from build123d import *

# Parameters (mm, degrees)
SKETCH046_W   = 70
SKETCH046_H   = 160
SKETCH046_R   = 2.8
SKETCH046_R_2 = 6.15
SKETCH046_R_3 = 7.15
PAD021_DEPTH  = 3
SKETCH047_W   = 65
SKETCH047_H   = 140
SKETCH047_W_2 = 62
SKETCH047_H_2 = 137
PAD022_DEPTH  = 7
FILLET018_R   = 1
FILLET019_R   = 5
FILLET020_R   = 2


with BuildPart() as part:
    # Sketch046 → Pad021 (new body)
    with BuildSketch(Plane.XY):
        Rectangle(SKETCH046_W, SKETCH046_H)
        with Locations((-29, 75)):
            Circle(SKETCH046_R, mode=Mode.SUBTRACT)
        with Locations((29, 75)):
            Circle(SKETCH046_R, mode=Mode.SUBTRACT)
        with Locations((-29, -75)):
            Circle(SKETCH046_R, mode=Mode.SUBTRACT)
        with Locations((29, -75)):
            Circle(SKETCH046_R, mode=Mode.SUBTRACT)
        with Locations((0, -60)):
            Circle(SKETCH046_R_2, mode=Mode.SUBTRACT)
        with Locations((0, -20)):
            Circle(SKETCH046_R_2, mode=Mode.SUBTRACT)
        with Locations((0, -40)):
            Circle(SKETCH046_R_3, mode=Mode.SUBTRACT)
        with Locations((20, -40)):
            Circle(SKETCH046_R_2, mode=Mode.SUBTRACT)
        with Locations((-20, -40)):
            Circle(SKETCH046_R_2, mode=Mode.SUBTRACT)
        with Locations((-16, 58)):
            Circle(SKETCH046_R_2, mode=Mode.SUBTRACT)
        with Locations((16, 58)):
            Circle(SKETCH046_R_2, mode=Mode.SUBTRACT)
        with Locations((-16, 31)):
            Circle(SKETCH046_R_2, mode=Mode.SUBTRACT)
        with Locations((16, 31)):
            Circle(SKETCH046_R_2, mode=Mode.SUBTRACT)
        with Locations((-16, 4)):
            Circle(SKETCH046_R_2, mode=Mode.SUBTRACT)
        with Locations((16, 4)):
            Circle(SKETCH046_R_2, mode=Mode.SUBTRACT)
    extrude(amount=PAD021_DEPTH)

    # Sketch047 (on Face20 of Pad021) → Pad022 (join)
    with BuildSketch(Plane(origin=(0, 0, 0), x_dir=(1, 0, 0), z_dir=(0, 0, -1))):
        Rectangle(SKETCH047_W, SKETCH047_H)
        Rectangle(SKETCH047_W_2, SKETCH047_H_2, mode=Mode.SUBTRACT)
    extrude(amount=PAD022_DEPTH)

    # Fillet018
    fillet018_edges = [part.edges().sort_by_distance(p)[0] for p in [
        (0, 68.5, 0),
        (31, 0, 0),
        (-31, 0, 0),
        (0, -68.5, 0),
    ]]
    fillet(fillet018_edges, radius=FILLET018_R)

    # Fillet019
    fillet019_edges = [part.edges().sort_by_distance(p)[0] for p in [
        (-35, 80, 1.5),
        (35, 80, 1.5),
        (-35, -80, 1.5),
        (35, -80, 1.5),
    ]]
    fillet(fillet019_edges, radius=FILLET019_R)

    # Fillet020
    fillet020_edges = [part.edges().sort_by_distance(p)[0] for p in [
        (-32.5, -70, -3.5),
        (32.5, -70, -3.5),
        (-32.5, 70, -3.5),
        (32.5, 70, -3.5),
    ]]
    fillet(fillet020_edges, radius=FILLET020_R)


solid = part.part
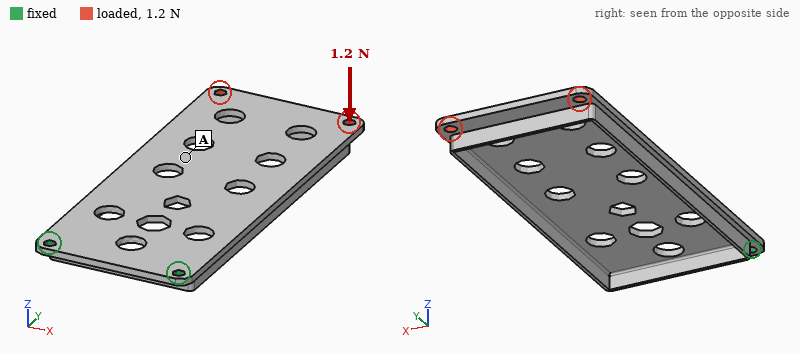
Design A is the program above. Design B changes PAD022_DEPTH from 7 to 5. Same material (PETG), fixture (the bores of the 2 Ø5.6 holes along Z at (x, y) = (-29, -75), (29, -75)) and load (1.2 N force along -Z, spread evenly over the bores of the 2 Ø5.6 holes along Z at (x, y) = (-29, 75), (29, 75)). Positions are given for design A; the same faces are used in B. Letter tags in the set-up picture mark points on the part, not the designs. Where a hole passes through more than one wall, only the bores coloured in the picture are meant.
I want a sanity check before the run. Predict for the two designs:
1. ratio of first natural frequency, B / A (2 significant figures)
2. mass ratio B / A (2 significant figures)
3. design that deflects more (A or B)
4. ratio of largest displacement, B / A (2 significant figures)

0.90
0.96
B
1.3
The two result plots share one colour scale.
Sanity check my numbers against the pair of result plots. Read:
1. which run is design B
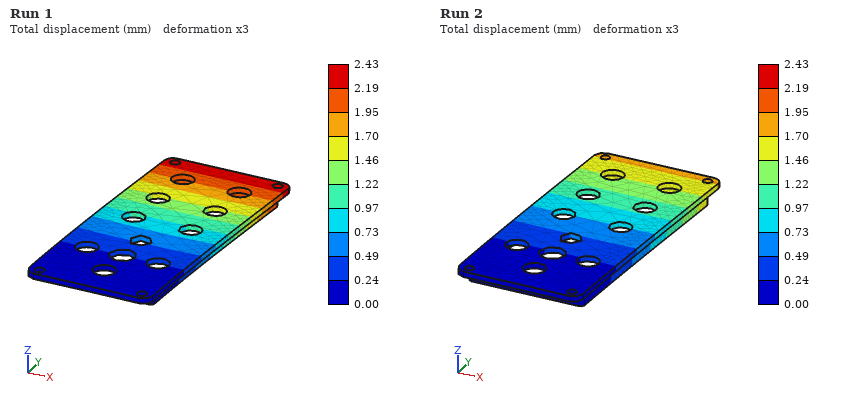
Run 1
